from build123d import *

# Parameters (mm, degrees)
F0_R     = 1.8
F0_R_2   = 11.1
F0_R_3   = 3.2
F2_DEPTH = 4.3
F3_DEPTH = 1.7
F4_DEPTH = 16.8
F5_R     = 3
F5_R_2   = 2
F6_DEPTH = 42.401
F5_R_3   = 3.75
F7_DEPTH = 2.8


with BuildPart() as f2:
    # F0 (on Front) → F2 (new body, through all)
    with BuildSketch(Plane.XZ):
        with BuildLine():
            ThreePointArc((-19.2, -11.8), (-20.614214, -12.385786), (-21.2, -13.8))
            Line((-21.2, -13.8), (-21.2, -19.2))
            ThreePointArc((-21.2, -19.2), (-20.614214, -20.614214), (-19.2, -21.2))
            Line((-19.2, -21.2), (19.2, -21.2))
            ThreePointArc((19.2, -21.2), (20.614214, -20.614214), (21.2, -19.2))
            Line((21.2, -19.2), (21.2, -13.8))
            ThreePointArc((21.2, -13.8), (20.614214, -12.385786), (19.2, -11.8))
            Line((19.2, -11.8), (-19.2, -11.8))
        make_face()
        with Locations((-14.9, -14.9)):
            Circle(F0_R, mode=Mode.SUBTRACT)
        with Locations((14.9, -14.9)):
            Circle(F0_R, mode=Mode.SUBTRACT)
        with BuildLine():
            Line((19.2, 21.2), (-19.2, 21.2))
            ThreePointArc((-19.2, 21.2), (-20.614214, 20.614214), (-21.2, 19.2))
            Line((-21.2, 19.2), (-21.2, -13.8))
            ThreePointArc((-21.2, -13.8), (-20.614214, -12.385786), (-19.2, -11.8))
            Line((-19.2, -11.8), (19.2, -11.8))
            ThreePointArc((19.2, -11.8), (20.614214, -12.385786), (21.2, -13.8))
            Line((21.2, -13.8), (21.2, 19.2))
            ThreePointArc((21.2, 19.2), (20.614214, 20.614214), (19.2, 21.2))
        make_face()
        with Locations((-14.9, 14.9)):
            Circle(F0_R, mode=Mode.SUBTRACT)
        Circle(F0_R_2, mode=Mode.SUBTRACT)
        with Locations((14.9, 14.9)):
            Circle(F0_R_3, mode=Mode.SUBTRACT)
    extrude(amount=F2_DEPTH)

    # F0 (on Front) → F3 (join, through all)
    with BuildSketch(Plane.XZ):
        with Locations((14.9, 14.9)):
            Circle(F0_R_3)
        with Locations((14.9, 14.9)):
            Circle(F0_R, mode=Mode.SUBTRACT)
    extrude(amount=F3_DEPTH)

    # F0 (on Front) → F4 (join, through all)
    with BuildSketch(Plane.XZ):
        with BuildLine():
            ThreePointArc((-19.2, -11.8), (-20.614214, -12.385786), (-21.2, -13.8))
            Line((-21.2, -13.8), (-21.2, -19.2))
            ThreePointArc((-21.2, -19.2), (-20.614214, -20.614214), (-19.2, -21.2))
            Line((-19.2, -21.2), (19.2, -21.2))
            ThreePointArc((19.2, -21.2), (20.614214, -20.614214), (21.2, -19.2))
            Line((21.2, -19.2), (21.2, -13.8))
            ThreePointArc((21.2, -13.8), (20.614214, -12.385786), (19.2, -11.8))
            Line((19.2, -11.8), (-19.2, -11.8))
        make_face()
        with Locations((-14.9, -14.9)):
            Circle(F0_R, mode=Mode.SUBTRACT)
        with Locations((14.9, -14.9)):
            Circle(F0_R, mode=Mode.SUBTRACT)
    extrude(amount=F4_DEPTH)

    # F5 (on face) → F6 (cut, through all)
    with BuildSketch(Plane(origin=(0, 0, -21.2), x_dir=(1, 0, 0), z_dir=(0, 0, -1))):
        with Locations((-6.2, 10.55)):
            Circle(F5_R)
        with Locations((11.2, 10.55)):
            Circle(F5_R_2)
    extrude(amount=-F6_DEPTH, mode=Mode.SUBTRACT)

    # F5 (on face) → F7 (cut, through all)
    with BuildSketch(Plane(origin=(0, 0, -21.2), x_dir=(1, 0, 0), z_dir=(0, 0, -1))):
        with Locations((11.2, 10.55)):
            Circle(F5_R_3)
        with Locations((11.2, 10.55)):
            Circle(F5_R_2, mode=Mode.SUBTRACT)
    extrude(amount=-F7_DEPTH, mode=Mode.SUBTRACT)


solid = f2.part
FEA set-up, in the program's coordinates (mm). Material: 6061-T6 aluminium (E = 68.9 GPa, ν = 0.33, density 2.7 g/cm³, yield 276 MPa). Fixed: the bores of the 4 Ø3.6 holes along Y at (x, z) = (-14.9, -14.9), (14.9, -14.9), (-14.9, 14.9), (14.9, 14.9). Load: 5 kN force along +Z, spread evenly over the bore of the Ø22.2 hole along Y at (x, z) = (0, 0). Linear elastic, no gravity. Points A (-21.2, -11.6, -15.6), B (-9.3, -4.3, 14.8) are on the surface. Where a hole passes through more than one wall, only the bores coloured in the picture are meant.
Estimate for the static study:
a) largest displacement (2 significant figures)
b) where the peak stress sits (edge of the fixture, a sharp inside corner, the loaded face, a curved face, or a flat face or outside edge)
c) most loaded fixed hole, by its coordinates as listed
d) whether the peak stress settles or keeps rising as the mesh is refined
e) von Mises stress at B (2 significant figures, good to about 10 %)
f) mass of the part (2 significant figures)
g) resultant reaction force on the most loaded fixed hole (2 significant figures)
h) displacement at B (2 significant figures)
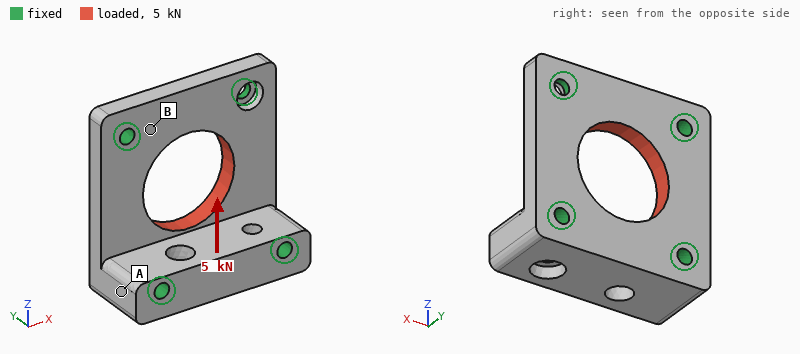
13 µm
edge of the fixture
(14.9, -14.9)
keeps rising
28 MPa
27 g
1.5 kN
4.8 µm
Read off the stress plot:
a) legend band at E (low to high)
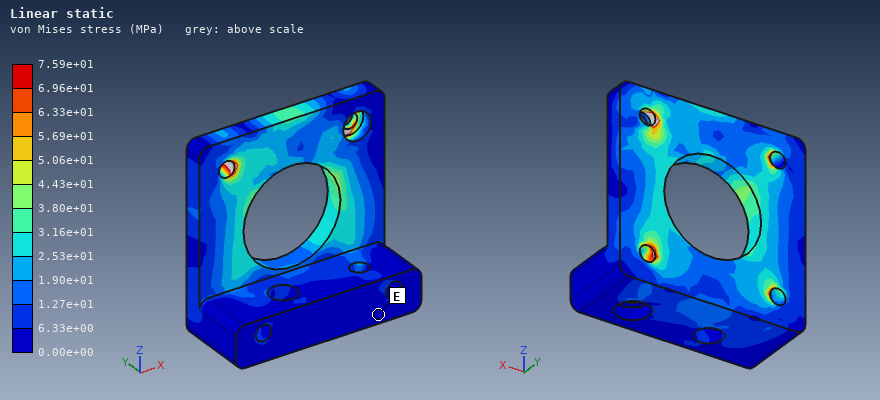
0.00e+00 to 6.33e+00 MPa
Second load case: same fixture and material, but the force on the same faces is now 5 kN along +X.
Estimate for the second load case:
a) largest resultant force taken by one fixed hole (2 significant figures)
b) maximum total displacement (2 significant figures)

1.4 kN
12 µm
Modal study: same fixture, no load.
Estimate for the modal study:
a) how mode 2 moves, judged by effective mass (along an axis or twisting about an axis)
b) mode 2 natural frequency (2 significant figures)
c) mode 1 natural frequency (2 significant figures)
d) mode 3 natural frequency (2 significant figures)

along Y
22 kHz
20 kHz
26 kHz
